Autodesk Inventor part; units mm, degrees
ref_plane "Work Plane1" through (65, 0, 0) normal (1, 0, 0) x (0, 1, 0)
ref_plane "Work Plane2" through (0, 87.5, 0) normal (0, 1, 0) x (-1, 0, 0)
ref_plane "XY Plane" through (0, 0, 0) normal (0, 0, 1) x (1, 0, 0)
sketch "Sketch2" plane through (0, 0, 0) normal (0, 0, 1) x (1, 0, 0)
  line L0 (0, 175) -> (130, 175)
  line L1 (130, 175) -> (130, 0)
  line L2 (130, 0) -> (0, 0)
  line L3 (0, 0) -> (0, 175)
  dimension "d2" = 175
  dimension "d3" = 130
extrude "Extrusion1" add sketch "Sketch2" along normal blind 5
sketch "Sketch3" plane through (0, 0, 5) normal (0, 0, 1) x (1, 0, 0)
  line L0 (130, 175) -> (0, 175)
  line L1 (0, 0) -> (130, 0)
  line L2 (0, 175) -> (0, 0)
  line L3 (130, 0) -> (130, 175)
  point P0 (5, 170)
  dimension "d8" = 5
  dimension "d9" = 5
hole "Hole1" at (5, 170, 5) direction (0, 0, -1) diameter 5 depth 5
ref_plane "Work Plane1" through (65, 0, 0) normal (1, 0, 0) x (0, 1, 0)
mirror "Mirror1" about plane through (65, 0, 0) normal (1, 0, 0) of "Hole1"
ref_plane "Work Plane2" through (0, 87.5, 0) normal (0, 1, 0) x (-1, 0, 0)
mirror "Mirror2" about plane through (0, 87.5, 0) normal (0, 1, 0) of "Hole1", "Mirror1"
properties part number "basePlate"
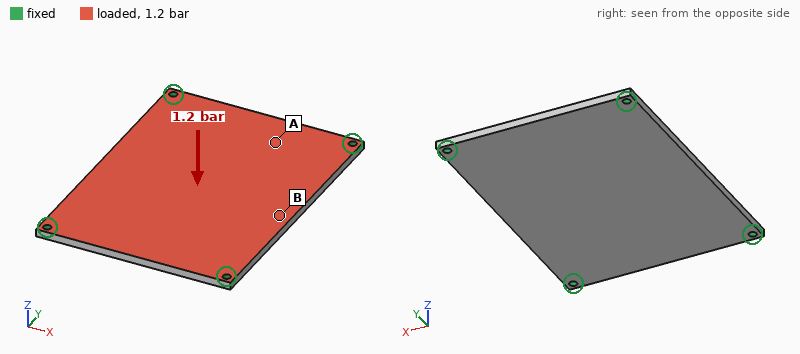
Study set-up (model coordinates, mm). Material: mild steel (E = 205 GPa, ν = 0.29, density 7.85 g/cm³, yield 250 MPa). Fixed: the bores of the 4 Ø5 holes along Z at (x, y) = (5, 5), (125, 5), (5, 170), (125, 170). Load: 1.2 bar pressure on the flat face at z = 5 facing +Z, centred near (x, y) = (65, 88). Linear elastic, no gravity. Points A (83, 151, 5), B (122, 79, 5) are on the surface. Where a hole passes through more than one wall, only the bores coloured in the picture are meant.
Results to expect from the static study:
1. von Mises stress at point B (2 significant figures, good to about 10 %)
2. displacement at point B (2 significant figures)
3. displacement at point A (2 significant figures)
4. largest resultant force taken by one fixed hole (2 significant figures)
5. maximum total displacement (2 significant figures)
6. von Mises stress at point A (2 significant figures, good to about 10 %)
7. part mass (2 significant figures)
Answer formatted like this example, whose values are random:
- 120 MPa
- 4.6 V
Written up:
- 49 MPa
- 0.19 mm
- 0.10 mm
- 680 N
- 0.23 mm
- 24 MPa
- 890 g
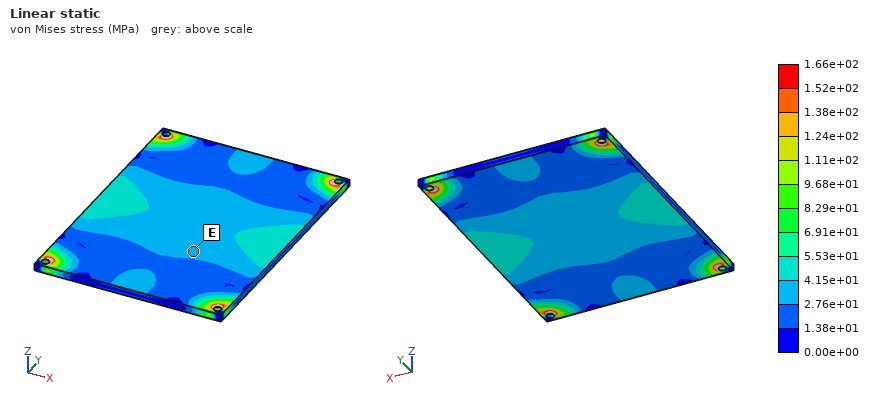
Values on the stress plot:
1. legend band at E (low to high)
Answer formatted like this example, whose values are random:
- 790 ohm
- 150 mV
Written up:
- 2.76e+01 to 4.15e+01 MPa
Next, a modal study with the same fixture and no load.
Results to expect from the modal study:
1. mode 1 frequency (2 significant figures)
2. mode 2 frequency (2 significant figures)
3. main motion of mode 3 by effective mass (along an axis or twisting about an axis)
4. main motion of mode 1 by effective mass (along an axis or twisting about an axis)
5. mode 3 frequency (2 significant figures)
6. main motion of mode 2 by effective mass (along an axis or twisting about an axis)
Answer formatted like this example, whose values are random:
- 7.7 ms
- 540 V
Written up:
- 680 Hz
- 1200 Hz
- twisting about X
- along Z
- 1600 Hz
- twisting about Y
